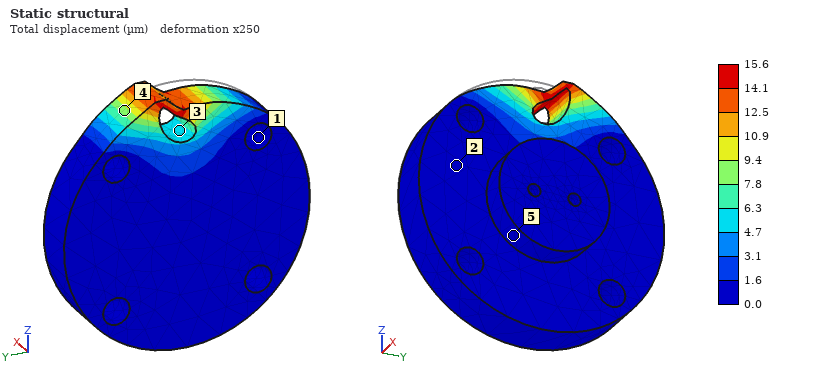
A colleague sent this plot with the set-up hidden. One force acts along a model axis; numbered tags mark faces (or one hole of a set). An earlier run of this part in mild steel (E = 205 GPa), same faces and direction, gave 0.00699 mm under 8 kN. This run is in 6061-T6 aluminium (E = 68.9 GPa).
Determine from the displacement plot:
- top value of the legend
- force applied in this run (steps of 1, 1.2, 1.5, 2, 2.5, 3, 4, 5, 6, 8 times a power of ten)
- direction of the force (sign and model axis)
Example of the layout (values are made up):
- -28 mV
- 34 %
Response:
- 15.6 µm
- 6 kN
- +Y
